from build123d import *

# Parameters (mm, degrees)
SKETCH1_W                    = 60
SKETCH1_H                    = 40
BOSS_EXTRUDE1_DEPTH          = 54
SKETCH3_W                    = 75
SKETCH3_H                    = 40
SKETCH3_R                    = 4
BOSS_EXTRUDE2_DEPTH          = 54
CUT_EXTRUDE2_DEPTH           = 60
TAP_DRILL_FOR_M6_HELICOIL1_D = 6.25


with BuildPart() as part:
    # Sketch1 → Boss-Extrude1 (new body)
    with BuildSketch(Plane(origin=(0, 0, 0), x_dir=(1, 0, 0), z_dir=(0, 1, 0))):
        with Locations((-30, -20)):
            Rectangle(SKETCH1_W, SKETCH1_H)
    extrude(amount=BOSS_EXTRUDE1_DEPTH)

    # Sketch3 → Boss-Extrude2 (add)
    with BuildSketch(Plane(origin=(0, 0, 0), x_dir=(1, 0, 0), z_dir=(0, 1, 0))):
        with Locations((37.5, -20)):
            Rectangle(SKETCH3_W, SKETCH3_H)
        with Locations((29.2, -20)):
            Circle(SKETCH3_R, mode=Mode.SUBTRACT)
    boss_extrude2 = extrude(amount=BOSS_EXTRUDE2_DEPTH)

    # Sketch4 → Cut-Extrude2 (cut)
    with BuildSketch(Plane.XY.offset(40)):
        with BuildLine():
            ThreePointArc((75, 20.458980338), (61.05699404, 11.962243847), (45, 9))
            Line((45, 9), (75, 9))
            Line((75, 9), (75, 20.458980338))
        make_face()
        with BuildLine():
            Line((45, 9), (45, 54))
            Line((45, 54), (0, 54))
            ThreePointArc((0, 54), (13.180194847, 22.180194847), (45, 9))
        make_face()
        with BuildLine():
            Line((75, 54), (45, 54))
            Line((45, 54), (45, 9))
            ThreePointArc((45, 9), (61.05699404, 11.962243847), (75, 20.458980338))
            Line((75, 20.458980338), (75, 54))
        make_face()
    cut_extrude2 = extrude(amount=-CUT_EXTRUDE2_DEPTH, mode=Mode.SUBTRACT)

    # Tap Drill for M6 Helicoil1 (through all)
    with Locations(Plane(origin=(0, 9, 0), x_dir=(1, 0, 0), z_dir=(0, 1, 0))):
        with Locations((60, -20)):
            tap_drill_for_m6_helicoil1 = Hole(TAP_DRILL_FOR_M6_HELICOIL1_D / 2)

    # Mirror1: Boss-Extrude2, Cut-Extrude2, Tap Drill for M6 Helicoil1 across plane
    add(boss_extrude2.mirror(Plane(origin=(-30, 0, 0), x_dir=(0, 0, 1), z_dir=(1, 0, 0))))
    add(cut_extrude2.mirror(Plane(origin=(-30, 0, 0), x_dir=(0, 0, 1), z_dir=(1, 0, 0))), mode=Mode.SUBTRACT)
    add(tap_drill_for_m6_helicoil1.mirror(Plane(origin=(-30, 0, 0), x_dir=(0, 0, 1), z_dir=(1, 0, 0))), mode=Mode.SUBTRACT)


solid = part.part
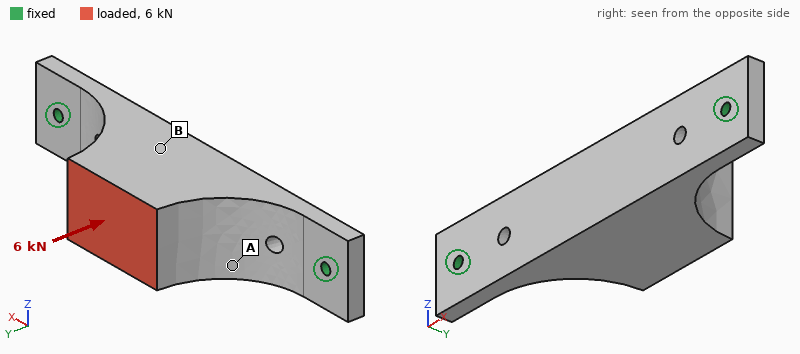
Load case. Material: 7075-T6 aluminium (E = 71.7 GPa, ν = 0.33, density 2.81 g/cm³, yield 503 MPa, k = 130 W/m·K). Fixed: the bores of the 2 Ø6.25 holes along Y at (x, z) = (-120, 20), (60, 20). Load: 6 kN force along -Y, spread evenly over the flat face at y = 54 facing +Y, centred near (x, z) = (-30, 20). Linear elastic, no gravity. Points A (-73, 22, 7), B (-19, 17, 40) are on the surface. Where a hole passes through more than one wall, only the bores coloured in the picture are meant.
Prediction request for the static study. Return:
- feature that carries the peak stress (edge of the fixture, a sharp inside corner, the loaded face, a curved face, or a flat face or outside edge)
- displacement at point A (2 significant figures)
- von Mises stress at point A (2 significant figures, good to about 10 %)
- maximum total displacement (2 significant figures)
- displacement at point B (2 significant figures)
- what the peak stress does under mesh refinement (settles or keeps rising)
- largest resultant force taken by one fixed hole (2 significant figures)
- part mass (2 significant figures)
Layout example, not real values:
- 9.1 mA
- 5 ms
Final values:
- edge of the fixture
- 0.10 mm
- 29 MPa
- 0.11 mm
- 0.11 mm
- keeps rising
- 4.7 kN
- 610 g
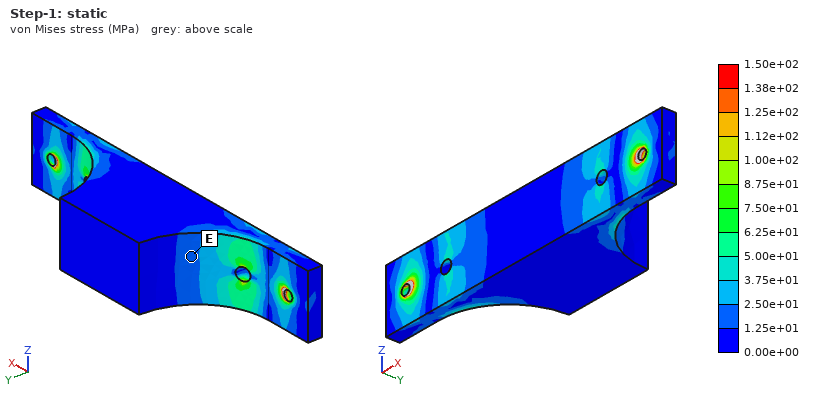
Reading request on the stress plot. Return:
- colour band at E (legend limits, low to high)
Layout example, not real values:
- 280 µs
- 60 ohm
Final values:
- 1.25e+01 to 2.50e+01 MPa
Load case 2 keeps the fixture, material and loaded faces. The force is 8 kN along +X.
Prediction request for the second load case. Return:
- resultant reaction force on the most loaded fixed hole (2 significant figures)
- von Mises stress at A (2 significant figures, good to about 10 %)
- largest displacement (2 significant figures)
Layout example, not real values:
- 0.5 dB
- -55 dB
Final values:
- 4.8 kN
- 26 MPa
- 77 µm
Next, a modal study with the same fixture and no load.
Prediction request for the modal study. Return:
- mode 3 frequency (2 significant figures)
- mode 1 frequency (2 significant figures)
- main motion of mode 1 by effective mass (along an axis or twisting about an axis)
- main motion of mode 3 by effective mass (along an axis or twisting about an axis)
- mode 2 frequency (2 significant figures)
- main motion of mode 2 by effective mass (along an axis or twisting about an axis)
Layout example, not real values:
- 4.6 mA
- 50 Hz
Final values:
- 3200 Hz
- 930 Hz
- along Z
- along Z
- 1600 Hz
- along Y
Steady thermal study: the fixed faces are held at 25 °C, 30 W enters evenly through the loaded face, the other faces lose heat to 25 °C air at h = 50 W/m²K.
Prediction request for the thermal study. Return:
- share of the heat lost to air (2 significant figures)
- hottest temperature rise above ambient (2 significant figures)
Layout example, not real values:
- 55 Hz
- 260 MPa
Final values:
- 38 %
- 14 K
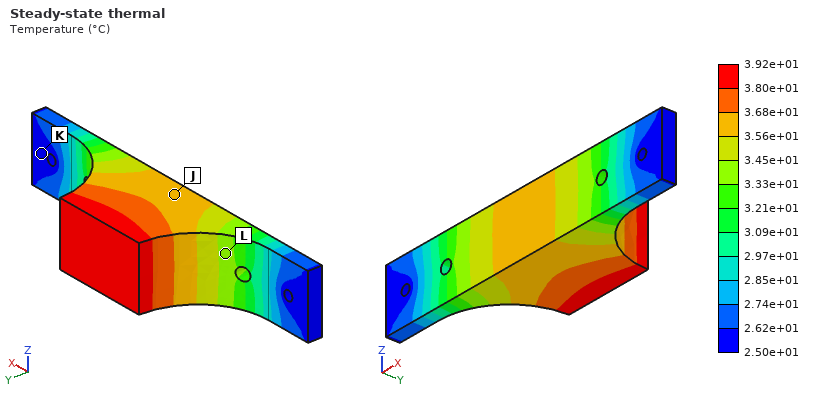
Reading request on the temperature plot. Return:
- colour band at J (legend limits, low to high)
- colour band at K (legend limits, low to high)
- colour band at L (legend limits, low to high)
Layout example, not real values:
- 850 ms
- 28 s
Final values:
- 3.56e+01 to 3.68e+01 °C
- 2.50e+01 to 2.62e+01 °C
- 3.33e+01 to 3.45e+01 °C
